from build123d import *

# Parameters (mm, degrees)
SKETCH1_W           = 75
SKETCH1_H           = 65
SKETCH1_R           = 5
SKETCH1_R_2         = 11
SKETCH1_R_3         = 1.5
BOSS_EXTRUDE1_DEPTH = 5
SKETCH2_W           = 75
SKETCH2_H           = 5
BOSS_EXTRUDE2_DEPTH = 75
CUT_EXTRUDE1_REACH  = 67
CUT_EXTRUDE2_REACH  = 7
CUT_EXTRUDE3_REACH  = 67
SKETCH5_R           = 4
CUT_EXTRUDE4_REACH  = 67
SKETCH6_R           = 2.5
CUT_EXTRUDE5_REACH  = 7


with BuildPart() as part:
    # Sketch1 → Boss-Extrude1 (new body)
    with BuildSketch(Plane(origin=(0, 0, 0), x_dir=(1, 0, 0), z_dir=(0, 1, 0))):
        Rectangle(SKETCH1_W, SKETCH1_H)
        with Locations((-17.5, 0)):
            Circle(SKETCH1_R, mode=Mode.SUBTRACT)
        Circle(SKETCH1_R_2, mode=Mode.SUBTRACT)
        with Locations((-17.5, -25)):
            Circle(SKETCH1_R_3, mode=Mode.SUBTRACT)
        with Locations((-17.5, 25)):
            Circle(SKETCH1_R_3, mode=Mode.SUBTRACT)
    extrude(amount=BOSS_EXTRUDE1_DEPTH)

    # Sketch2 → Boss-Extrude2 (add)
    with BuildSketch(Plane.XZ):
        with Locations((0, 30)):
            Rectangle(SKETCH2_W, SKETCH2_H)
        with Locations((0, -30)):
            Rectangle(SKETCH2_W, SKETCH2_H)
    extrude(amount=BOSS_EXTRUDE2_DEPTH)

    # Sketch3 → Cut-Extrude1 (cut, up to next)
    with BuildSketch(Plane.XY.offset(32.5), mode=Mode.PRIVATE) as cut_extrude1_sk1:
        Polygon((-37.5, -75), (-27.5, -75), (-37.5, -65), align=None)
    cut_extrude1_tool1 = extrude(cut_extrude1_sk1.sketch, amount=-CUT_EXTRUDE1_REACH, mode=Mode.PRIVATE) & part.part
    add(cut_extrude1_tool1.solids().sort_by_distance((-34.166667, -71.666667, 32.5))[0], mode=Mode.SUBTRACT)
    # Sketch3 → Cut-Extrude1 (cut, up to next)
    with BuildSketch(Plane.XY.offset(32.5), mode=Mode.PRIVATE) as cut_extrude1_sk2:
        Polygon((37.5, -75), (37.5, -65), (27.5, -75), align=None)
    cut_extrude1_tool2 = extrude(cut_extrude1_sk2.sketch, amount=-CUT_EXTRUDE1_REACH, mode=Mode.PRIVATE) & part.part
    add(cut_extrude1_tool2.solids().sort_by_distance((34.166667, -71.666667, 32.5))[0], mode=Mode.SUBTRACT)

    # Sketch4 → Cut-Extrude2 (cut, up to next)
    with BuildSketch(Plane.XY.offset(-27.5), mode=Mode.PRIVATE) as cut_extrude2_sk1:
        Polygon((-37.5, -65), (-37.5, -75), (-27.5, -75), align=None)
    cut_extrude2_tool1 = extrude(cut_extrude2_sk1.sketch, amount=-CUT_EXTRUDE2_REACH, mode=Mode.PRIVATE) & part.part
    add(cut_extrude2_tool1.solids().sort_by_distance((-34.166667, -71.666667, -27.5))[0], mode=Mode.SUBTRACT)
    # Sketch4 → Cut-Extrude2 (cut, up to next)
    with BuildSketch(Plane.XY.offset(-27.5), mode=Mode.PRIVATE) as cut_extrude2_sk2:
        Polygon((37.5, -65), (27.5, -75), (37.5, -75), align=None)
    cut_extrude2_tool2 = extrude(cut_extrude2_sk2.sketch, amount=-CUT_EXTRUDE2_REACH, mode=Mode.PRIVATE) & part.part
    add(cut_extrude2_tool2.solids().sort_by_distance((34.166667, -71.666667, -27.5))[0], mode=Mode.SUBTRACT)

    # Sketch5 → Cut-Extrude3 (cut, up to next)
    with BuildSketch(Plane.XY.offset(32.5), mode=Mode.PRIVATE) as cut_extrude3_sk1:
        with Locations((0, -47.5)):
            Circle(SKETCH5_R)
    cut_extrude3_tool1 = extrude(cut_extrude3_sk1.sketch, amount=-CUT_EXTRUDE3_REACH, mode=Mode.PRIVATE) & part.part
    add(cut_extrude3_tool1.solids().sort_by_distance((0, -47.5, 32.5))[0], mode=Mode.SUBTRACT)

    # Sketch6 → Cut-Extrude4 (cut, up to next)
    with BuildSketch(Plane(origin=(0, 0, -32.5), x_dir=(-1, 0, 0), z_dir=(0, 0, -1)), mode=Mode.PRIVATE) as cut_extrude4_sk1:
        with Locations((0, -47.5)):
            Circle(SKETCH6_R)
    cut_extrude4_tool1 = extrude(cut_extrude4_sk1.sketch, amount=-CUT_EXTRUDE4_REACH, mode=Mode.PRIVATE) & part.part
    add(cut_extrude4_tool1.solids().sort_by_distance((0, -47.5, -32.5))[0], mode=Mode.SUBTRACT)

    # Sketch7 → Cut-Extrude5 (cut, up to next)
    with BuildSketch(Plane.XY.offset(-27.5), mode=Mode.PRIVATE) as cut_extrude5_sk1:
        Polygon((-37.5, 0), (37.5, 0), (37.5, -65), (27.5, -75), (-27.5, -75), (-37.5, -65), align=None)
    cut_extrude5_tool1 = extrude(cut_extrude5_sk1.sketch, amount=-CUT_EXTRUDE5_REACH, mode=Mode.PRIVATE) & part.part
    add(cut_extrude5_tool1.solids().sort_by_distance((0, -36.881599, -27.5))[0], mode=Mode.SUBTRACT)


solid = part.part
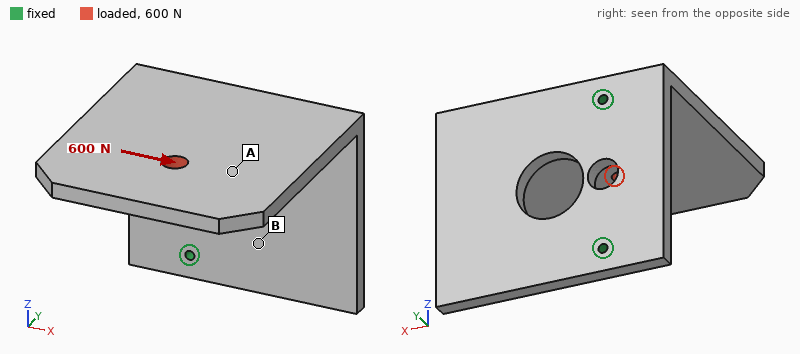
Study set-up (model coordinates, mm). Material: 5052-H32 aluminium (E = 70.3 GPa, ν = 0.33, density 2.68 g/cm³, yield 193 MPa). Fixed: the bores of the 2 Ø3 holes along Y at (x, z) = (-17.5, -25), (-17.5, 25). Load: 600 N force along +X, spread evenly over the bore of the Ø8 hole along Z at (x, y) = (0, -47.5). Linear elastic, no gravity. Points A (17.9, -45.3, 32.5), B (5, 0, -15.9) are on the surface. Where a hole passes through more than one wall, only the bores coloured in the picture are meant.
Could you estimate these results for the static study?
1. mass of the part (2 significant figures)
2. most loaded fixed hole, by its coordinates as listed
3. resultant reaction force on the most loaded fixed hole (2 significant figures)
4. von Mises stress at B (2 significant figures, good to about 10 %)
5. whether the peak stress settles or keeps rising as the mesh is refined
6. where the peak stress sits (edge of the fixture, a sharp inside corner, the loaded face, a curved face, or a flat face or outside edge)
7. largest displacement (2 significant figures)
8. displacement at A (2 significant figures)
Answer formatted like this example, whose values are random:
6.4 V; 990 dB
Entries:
130 g; (-17.5, 25); 640 N; 23 MPa; keeps rising; edge of the fixture; 0.64 mm; 0.42 mm
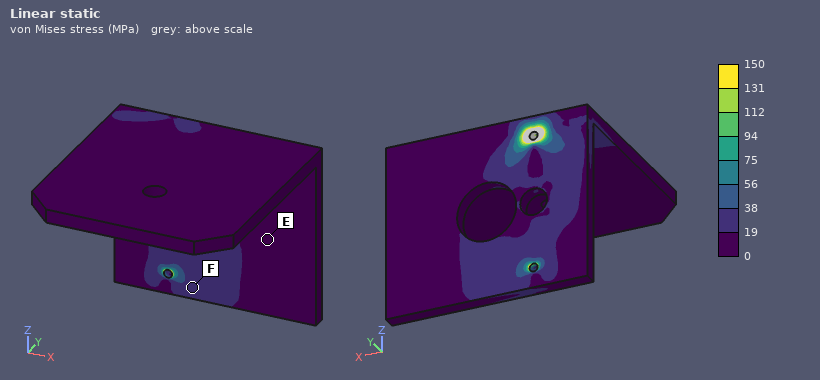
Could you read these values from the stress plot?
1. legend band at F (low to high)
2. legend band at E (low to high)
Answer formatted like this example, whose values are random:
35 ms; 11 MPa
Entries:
19 to 38 MPa; 0 to 19 MPa
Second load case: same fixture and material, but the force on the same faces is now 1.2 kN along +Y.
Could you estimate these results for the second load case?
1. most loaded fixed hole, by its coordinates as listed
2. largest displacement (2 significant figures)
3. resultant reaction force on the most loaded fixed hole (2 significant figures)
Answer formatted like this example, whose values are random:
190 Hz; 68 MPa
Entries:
(-17.5, 25); 0.48 mm; 1.2 kN
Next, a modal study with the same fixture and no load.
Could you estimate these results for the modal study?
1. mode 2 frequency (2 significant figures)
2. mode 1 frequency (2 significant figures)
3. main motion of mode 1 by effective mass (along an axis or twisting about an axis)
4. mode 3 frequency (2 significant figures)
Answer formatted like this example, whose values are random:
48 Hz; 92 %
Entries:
690 Hz; 550 Hz; along Z; 1600 Hz
